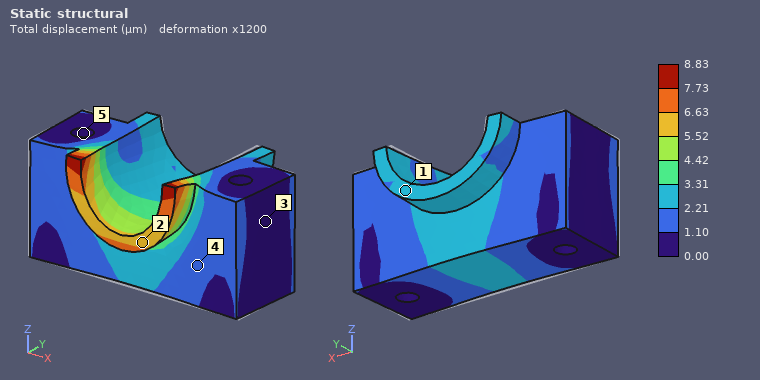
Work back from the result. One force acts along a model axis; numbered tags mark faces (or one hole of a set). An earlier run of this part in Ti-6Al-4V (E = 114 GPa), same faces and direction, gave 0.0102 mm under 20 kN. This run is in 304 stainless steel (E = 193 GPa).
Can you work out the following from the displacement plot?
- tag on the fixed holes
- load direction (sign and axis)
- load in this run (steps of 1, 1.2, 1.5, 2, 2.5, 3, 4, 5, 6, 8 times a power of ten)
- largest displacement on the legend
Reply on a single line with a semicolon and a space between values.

5; +Y; 30 kN; 8.83 µm
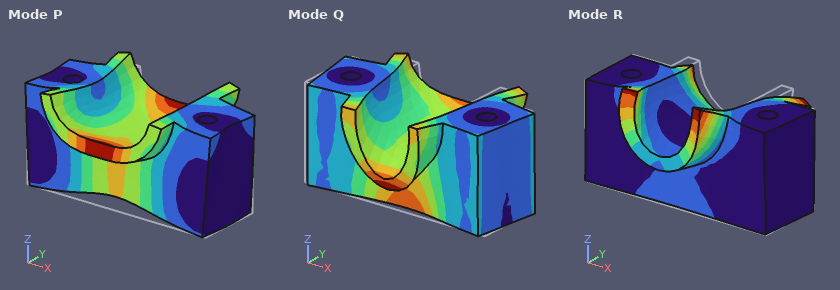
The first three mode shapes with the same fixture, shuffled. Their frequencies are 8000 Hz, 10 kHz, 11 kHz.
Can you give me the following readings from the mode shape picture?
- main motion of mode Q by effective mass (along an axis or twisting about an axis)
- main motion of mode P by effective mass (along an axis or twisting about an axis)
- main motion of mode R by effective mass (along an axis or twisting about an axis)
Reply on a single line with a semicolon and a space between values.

along Y; along Z; twisting about X
